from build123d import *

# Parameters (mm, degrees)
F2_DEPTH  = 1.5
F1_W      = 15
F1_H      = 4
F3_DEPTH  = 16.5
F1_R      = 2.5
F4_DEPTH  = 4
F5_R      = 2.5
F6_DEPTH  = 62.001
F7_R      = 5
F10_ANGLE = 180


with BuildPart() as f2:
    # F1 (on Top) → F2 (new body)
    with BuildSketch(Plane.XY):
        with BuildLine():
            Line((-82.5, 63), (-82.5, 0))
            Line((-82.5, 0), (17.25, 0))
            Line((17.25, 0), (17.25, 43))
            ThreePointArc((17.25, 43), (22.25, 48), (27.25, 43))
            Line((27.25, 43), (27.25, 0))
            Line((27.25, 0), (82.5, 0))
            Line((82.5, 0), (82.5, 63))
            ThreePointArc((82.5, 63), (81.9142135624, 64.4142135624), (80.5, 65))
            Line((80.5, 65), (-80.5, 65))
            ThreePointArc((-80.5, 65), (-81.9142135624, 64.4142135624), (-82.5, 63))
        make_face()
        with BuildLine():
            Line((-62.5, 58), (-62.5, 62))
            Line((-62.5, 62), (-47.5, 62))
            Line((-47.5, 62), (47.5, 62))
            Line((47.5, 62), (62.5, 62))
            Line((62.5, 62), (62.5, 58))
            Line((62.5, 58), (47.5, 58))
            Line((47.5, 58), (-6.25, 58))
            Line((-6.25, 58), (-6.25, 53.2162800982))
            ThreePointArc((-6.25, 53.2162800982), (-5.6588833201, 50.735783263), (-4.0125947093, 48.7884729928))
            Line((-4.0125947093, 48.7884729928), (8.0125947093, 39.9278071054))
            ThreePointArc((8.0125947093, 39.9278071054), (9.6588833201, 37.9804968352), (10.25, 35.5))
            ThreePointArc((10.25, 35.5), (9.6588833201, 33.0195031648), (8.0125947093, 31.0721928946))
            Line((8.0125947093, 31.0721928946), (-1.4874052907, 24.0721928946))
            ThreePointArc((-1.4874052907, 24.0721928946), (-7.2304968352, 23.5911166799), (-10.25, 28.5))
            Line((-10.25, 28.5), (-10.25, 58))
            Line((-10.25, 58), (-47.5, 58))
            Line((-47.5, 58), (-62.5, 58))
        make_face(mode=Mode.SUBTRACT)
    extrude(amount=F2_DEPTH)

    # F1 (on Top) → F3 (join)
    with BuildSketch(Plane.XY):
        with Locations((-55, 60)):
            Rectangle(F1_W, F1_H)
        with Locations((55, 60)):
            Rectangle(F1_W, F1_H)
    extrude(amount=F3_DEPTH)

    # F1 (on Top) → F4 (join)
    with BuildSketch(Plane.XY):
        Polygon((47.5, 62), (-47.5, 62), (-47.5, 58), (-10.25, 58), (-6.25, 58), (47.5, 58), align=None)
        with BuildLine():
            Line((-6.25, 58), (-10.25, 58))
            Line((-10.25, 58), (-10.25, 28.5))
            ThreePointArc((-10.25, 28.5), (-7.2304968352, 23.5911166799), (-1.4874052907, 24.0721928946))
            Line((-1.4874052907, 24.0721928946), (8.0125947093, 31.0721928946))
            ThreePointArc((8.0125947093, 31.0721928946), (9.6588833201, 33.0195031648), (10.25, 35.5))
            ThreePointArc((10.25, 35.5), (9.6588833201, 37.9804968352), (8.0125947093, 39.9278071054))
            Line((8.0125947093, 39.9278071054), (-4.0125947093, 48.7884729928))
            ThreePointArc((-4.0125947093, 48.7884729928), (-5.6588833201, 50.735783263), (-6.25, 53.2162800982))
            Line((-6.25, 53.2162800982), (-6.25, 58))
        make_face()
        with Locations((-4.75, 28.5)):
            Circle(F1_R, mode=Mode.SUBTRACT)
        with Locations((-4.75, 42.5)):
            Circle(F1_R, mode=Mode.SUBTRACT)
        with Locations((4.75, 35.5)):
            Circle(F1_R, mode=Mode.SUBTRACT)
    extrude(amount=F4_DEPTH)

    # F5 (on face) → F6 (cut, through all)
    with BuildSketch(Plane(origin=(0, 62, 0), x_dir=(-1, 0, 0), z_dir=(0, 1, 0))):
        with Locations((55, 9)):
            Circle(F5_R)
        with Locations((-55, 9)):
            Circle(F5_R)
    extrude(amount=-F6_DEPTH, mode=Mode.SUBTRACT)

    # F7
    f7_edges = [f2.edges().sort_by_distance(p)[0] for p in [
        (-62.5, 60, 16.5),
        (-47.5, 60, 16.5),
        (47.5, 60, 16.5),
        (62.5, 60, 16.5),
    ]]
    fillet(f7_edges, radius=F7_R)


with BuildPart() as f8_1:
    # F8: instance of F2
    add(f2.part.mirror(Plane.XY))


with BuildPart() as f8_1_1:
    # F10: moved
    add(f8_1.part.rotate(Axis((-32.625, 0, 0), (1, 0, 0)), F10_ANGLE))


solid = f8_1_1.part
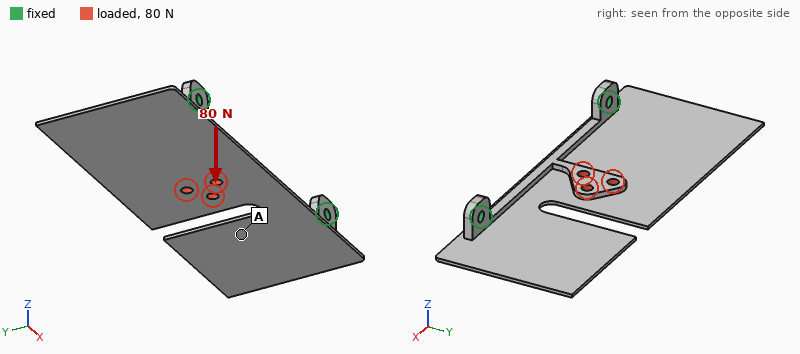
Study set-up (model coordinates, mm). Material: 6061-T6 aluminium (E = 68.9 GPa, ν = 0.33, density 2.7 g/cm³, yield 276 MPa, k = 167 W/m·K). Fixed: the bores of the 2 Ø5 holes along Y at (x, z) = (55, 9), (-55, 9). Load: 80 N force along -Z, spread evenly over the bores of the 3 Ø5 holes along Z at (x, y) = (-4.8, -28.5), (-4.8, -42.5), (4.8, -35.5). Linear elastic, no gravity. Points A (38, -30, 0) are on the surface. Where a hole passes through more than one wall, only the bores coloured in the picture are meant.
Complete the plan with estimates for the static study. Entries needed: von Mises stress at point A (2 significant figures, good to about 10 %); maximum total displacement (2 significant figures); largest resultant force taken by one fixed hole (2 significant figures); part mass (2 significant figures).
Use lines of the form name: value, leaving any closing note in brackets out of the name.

von Mises stress at point A: 7.0 MPa
maximum total displacement: 1.3 mm
largest resultant force taken by one fixed hole: 54 N
part mass: 50 g
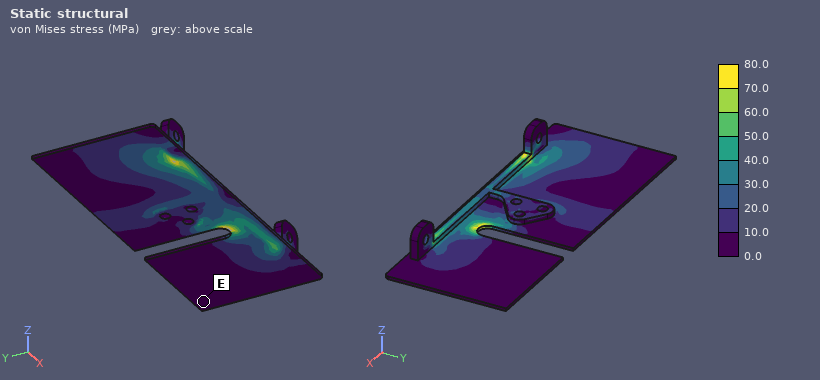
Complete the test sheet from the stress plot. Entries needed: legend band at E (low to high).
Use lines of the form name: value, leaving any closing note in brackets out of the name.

legend band at E: 0.0 to 10.0 MPa
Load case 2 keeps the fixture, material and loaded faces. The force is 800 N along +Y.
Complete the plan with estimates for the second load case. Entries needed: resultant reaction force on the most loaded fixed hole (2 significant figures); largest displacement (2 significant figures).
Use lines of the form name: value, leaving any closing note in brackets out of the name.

resultant reaction force on the most loaded fixed hole: 520 N
largest displacement: 0.50 mm
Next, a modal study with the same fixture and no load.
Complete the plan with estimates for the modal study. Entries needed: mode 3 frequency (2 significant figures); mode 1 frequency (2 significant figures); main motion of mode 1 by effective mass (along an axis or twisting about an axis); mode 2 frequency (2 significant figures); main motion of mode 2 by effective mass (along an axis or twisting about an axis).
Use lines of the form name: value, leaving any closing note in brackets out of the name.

mode 3 frequency: 560 Hz
mode 1 frequency: 310 Hz
main motion of mode 1 by effective mass: along Z
mode 2 frequency: 350 Hz
main motion of mode 2 by effective mass: twisting about Y
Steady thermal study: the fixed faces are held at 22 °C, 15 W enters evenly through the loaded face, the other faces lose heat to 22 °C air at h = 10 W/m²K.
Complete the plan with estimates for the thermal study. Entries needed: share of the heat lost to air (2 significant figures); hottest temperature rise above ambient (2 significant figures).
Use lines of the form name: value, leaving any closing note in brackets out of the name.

share of the heat lost to air: 25 %
hottest temperature rise above ambient: 41 K
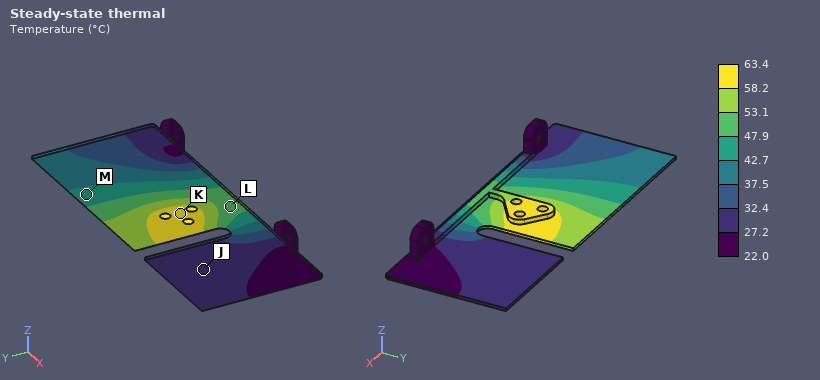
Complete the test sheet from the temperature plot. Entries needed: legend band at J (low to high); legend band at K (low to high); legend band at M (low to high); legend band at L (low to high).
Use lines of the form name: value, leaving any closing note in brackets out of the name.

legend band at J: 27.2 to 32.4 °C
legend band at K: 58.2 to 63.4 °C
legend band at M: 42.7 to 47.9 °C
legend band at L: 47.9 to 53.1 °C
